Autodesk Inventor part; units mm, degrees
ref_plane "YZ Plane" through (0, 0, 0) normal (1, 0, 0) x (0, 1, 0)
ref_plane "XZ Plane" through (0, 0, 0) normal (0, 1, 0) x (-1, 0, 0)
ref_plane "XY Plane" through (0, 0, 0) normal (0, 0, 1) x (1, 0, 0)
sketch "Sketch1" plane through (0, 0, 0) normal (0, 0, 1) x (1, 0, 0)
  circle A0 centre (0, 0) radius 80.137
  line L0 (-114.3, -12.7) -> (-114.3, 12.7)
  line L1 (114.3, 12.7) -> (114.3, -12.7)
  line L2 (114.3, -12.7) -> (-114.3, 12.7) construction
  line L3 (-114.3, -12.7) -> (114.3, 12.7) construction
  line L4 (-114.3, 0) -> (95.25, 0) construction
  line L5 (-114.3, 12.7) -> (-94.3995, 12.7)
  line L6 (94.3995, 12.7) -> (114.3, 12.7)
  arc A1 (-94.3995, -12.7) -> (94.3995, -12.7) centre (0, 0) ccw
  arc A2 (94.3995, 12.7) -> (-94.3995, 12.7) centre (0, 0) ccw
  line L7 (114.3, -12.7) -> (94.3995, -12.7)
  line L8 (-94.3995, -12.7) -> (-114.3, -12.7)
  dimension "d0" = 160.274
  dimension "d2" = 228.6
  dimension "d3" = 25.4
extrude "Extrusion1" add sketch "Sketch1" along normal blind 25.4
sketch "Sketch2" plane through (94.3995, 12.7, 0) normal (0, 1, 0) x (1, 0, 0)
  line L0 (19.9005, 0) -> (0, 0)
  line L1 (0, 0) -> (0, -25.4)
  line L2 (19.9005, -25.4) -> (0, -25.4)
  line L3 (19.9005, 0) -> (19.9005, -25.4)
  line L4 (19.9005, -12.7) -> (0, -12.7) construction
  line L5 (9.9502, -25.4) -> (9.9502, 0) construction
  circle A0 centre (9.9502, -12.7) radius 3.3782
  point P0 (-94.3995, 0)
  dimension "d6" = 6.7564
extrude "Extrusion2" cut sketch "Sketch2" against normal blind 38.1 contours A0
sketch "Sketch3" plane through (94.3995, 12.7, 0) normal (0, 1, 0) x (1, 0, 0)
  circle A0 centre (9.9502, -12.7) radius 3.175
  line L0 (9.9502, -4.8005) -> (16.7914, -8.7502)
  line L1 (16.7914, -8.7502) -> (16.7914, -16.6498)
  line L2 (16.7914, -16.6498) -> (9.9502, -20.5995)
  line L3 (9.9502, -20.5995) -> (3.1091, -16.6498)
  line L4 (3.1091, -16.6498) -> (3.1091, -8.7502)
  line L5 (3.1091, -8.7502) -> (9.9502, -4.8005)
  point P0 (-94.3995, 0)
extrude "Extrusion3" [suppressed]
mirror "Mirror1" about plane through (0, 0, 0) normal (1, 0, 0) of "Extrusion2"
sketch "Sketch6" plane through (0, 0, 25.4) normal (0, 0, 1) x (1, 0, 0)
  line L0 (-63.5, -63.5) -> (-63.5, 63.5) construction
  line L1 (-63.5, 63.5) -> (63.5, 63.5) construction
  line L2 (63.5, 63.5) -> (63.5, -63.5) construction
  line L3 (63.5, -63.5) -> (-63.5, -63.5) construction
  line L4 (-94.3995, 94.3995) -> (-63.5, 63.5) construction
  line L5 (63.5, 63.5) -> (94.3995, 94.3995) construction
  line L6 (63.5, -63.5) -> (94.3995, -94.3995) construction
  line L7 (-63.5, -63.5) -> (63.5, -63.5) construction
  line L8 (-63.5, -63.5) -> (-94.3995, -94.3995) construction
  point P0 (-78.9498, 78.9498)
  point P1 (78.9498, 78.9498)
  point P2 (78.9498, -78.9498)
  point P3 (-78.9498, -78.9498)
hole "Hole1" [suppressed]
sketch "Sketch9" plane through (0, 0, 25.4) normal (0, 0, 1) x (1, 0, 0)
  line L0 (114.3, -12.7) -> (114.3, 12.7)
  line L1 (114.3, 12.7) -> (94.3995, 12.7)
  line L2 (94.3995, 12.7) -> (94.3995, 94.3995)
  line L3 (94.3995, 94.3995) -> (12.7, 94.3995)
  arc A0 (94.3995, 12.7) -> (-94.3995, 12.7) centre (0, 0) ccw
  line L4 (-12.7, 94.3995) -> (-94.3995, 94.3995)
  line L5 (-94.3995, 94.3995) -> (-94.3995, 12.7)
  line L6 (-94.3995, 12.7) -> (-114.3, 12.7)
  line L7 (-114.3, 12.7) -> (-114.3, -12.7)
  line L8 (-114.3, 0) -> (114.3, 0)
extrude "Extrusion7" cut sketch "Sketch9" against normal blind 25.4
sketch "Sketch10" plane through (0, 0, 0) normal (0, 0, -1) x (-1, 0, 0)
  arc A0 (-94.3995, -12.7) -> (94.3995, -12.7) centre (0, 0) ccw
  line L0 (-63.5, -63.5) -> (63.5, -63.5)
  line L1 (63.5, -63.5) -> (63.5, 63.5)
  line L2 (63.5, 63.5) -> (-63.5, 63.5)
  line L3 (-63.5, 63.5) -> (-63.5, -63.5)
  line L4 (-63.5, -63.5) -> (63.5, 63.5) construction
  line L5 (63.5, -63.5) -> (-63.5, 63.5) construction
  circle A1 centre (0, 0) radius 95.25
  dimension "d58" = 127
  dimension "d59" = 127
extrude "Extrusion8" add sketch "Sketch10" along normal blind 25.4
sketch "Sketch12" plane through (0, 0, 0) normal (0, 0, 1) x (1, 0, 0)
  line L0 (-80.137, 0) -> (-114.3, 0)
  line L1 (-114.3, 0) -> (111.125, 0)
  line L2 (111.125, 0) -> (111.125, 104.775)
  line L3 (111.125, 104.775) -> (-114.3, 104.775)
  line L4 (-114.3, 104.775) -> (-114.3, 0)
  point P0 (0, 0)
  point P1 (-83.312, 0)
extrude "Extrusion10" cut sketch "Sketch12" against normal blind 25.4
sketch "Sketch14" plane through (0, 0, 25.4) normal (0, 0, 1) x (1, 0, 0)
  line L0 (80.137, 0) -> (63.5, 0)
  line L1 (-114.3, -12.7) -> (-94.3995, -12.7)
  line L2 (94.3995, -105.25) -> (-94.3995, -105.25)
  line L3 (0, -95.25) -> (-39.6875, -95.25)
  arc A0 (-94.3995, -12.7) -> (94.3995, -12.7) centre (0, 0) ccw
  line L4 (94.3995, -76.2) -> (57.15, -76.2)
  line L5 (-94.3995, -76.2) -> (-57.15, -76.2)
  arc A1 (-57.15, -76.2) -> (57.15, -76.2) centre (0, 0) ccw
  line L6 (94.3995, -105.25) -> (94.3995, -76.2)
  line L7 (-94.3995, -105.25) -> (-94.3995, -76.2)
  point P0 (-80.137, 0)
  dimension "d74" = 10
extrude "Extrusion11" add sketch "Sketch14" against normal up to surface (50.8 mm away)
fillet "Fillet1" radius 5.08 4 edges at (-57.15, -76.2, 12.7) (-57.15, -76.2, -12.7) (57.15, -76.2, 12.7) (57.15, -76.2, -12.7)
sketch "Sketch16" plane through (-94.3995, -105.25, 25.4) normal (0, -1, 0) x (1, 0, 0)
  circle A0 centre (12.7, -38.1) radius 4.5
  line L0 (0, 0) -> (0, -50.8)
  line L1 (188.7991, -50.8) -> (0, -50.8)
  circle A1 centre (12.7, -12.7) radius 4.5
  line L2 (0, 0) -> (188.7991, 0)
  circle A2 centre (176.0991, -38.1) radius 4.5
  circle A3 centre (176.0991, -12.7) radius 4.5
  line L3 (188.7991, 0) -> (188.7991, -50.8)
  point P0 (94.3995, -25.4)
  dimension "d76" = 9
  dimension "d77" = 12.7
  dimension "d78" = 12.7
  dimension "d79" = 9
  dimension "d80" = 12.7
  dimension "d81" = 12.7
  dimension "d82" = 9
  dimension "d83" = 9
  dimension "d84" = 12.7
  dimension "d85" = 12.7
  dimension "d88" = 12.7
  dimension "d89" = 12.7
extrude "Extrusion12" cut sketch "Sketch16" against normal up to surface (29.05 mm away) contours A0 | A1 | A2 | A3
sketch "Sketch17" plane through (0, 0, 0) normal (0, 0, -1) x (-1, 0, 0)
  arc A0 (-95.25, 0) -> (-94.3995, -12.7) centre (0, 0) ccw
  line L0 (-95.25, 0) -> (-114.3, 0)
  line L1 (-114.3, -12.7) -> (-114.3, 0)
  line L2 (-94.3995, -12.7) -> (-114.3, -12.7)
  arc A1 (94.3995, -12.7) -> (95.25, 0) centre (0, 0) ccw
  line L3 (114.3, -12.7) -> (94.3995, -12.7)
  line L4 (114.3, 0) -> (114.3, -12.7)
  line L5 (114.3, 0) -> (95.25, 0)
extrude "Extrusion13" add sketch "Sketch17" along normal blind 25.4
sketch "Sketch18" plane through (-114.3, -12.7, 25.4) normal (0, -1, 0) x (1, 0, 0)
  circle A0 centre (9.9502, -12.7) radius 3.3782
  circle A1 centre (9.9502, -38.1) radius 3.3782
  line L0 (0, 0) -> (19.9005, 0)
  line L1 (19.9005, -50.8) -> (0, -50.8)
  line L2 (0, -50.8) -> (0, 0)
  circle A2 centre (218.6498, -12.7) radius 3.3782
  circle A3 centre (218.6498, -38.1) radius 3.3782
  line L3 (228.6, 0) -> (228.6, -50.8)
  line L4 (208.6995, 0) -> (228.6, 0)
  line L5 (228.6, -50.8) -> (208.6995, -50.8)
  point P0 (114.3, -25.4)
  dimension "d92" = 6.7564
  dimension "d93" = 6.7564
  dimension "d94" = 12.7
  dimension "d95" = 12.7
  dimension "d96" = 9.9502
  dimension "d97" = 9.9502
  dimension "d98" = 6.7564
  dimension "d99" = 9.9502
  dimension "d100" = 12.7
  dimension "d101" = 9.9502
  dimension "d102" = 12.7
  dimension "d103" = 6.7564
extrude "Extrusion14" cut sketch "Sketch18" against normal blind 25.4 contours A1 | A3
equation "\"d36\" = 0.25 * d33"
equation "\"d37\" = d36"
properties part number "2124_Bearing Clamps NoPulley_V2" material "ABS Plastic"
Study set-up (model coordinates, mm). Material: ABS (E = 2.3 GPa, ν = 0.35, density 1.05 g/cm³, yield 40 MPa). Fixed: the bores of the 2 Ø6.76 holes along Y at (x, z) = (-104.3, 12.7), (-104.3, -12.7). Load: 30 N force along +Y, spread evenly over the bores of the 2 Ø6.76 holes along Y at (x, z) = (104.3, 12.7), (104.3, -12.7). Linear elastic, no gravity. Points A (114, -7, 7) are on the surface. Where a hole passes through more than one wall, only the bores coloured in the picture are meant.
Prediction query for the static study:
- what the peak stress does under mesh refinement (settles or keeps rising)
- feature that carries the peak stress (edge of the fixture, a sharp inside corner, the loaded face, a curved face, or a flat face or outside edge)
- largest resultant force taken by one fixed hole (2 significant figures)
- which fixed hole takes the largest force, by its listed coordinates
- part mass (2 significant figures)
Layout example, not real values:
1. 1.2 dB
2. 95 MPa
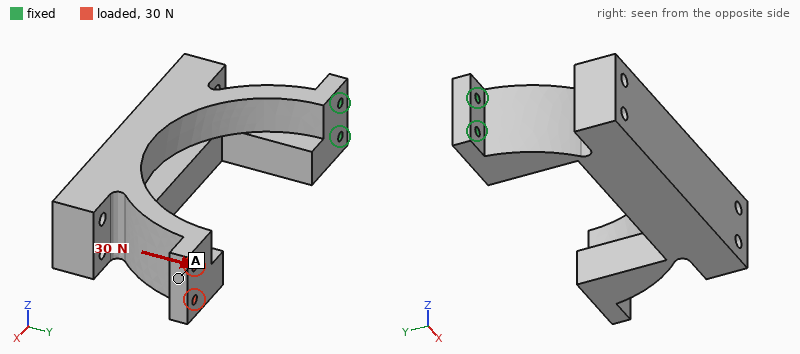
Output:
1. keeps rising
2. edge of the fixture
3. 22 N
4. (-104.3, 12.7)
5. 510 g
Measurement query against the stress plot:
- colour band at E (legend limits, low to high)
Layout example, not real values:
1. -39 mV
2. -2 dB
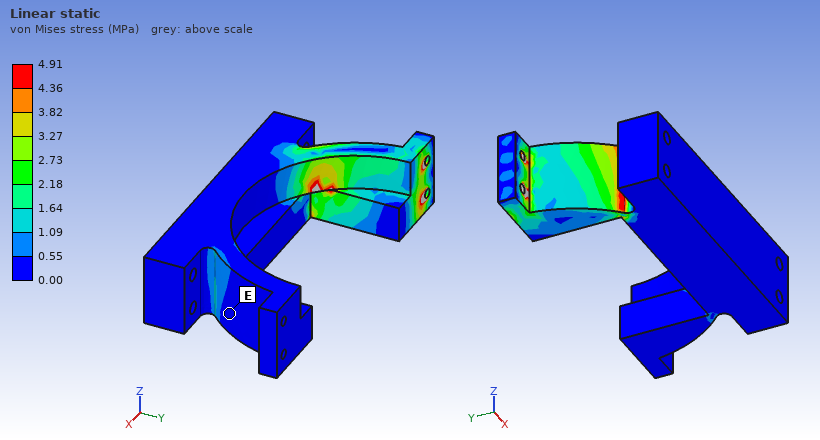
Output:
1. 0.00 to 0.55 MPa
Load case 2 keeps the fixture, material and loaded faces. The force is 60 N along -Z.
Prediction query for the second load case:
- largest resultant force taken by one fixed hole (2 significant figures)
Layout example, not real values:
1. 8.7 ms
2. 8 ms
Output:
1. 430 N
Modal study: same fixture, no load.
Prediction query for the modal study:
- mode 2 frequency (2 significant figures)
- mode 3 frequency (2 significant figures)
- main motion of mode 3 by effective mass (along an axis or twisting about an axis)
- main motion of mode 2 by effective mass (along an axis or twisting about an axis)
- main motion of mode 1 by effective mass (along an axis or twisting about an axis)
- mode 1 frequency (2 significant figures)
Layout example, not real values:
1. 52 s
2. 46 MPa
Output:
1. 71 Hz
2. 180 Hz
3. along X
4. along Z
5. along Y
6. 39 Hz
